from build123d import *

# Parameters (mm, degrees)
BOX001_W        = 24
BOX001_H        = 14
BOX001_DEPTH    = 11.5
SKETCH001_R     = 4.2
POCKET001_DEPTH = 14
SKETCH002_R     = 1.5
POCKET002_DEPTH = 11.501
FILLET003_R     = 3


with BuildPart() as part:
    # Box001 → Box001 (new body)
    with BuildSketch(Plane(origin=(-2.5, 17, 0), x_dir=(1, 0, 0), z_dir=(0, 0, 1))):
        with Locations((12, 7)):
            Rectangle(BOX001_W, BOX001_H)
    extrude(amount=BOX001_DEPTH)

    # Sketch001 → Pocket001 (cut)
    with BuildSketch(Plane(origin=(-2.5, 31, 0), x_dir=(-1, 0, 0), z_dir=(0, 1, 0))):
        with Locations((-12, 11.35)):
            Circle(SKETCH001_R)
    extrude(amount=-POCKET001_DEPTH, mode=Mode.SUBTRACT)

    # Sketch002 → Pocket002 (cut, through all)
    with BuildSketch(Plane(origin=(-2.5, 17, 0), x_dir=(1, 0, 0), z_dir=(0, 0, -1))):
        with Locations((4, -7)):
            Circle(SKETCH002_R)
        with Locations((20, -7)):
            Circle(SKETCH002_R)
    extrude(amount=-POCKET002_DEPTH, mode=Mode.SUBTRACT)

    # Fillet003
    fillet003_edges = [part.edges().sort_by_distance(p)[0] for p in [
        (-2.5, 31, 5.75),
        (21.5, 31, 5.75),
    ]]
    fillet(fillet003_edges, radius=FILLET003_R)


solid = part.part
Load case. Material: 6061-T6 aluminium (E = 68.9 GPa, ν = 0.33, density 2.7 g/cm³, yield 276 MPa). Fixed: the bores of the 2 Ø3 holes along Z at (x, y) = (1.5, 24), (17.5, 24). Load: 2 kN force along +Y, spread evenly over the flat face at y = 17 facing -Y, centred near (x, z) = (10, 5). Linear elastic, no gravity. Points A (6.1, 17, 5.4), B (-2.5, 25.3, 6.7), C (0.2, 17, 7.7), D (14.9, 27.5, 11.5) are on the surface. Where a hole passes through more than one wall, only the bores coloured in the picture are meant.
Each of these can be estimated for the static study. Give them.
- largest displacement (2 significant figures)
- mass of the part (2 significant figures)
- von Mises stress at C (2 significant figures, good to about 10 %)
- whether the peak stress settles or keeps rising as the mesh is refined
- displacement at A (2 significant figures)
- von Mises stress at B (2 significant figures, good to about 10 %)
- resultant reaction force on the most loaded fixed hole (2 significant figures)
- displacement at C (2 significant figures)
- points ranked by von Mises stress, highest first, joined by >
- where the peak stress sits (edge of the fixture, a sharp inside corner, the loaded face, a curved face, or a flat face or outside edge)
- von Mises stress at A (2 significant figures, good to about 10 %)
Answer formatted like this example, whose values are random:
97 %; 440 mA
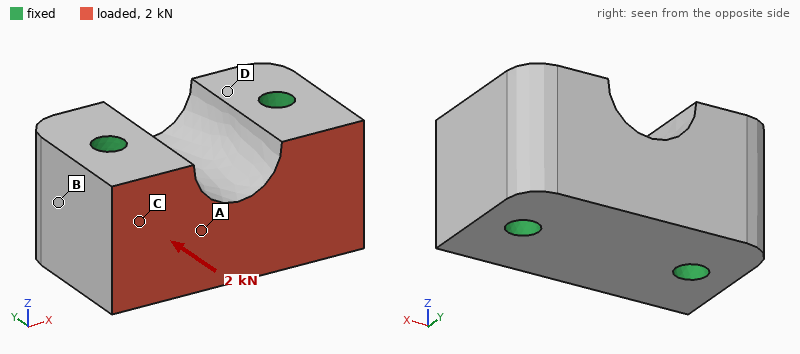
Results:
1.6 µm; 8.8 g; 9.2 MPa; keeps rising; 1.2 µm; 4.1 MPa; 1.0 kN; 0.80 µm; C > A > B > D; edge of the fixture; 7.0 MPa
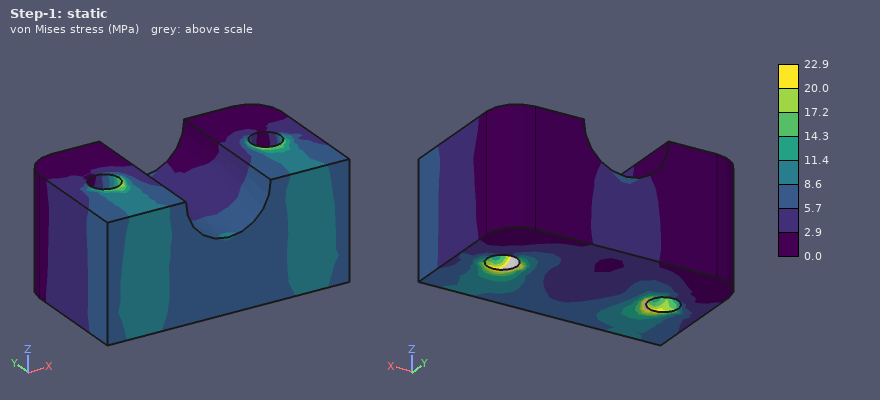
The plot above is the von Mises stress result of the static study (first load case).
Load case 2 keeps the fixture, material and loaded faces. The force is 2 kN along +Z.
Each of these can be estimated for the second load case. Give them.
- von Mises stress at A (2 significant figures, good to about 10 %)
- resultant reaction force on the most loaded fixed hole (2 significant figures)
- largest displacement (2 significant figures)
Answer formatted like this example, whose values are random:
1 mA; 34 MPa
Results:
19 MPa; 1.0 kN; 6.1 µm
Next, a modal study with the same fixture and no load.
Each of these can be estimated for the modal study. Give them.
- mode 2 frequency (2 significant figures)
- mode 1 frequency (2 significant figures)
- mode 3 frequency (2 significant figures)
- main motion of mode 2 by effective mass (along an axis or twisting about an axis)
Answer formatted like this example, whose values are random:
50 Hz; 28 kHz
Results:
77 kHz; 72 kHz; 83 kHz; along Z
